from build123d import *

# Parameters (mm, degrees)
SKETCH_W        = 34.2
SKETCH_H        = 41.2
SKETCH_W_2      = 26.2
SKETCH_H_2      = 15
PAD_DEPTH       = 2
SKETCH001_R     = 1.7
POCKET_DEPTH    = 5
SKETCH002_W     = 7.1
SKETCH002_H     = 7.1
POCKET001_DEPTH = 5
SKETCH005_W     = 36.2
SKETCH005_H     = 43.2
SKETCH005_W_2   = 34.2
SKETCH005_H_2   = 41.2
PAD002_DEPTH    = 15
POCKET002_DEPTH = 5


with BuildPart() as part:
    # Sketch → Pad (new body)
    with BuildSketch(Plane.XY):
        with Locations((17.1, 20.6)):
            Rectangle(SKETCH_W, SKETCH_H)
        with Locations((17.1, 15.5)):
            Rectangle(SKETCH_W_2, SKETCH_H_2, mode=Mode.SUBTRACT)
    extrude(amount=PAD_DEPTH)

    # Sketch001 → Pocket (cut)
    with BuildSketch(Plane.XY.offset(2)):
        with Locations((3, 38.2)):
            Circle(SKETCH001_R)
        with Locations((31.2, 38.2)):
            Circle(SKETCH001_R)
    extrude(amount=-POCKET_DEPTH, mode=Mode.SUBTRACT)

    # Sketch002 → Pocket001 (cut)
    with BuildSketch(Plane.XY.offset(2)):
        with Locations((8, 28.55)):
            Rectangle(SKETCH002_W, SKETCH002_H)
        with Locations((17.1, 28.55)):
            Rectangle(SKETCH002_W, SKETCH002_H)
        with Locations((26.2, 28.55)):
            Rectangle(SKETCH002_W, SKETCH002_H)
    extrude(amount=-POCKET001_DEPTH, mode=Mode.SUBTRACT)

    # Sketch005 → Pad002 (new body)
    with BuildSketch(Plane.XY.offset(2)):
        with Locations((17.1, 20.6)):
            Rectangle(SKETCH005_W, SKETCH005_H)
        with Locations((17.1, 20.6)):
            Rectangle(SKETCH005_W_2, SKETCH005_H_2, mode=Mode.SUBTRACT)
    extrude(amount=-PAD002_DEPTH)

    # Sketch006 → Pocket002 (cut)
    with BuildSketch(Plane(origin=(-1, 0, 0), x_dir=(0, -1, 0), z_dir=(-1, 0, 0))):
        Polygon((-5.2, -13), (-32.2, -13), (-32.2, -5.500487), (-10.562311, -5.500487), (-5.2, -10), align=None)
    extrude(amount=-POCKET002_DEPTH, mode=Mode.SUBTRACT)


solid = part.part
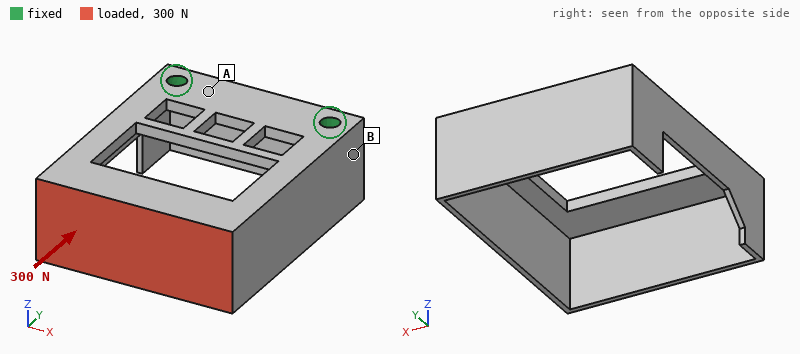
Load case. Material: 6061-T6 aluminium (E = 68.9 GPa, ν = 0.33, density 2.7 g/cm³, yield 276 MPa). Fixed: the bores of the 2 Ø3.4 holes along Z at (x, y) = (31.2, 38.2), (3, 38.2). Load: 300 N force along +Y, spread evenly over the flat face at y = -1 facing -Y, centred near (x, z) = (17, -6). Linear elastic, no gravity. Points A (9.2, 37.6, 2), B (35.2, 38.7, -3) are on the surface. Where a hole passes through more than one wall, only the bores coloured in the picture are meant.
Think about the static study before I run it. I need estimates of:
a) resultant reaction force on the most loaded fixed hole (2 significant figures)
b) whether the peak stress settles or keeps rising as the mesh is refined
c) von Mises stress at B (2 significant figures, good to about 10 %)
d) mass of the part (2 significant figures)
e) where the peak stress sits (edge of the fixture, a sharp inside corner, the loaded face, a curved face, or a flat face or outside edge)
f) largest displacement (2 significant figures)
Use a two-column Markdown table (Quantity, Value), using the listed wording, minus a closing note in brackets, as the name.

| Quantity | Value |
|---|---|
| resultant reaction force on the most loaded fixed hole | 160 N |
| whether the peak stress settles or keeps rising as the mesh is refined | keeps rising |
| von Mises stress at B | 26 MPa |
| mass of the part | 10 g |
| where the peak stress sits | edge of the fixture |
| largest displacement | 0.35 mm |
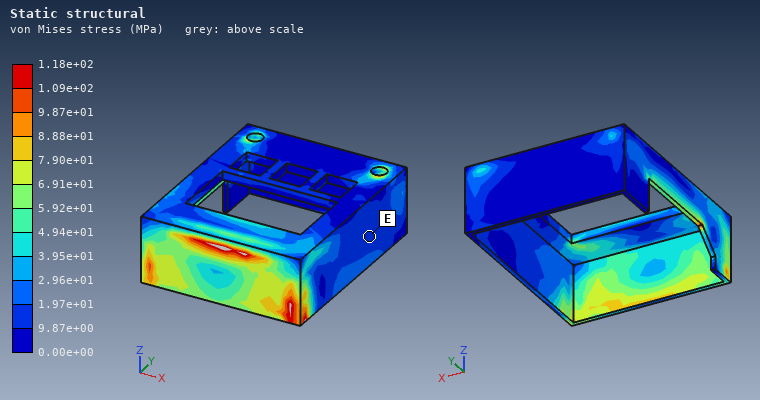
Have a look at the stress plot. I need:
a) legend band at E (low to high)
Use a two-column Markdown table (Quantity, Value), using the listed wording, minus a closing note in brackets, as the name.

| Quantity | Value |
|---|---|
| legend band at E | 9.87e+00 to 1.97e+01 MPa |
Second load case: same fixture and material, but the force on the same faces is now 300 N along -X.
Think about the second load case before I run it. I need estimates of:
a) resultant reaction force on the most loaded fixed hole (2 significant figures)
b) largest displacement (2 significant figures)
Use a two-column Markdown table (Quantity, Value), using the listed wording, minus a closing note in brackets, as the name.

| Quantity | Value |
|---|---|
| resultant reaction force on the most loaded fixed hole | 390 N |
| largest displacement | 0.57 mm |
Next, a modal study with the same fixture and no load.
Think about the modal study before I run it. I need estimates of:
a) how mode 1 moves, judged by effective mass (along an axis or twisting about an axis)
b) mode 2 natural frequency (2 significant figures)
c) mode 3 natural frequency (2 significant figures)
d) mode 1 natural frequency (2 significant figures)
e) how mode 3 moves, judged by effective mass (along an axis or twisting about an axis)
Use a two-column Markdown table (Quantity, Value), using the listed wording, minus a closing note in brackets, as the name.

| Quantity | Value |
|---|---|
| how mode 1 moves, judged by effective mass | along Z |
| mode 2 natural frequency | 2100 Hz |
| mode 3 natural frequency | 3700 Hz |
| mode 1 natural frequency | 1600 Hz |
| how mode 3 moves, judged by effective mass | along X |
